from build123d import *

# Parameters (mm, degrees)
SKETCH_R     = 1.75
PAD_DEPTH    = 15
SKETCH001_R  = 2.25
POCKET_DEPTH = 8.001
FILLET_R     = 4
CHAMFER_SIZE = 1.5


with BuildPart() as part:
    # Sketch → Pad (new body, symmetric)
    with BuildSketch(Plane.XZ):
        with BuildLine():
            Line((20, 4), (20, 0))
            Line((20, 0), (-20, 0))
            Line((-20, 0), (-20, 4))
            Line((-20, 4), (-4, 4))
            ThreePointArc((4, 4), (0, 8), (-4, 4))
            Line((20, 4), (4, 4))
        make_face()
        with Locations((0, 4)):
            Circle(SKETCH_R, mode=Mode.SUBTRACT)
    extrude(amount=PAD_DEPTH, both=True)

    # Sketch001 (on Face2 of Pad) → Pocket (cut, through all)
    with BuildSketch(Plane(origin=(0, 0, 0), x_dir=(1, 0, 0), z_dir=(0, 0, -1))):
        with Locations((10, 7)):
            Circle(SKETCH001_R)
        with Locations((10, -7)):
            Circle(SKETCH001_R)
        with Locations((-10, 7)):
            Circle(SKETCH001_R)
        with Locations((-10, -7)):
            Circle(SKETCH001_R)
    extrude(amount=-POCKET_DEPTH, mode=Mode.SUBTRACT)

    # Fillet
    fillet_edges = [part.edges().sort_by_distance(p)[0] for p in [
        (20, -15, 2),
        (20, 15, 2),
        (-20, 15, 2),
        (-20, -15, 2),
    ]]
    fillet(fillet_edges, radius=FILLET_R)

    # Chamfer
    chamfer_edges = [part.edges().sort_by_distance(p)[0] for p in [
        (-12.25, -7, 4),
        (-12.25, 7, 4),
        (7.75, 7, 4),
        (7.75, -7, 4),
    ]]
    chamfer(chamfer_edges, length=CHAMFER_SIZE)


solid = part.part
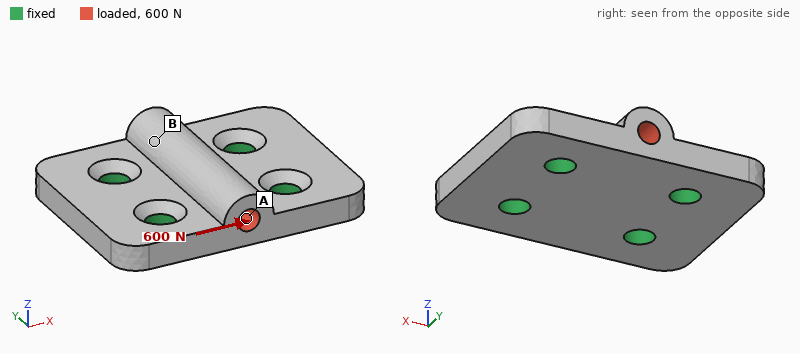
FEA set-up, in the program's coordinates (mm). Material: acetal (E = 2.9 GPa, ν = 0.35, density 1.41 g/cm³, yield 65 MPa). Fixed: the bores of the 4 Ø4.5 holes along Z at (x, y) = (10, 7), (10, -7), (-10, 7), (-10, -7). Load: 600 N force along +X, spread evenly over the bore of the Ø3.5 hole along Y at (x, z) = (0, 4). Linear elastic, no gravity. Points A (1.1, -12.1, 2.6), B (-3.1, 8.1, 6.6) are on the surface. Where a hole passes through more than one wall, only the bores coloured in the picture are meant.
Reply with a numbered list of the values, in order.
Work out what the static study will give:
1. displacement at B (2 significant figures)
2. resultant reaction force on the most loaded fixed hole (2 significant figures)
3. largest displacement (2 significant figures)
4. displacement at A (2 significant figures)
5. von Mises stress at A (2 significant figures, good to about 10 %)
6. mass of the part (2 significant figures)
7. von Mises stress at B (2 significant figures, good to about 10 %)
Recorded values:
1. 17 µm
2. 160 N
3. 18 µm
4. 9.7 µm
5. 3.6 MPa
6. 6.9 g
7. 1.7 MPa
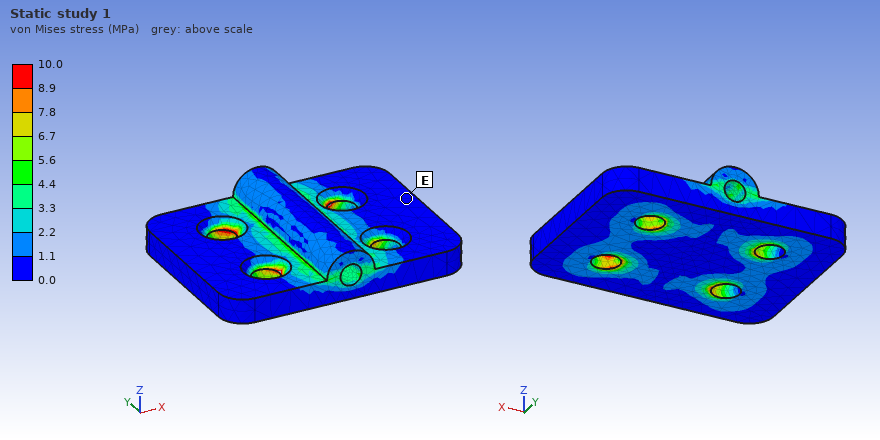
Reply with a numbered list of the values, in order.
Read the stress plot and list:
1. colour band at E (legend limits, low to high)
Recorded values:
1. 0.0 to 1.1 MPa
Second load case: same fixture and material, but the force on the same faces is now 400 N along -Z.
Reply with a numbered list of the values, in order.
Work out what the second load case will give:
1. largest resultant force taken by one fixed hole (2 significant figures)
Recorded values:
1. 110 N
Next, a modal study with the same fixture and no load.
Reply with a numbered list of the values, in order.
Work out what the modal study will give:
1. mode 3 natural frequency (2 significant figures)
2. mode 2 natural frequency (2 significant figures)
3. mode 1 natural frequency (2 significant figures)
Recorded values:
1. 8900 Hz
2. 7900 Hz
3. 7600 Hz
